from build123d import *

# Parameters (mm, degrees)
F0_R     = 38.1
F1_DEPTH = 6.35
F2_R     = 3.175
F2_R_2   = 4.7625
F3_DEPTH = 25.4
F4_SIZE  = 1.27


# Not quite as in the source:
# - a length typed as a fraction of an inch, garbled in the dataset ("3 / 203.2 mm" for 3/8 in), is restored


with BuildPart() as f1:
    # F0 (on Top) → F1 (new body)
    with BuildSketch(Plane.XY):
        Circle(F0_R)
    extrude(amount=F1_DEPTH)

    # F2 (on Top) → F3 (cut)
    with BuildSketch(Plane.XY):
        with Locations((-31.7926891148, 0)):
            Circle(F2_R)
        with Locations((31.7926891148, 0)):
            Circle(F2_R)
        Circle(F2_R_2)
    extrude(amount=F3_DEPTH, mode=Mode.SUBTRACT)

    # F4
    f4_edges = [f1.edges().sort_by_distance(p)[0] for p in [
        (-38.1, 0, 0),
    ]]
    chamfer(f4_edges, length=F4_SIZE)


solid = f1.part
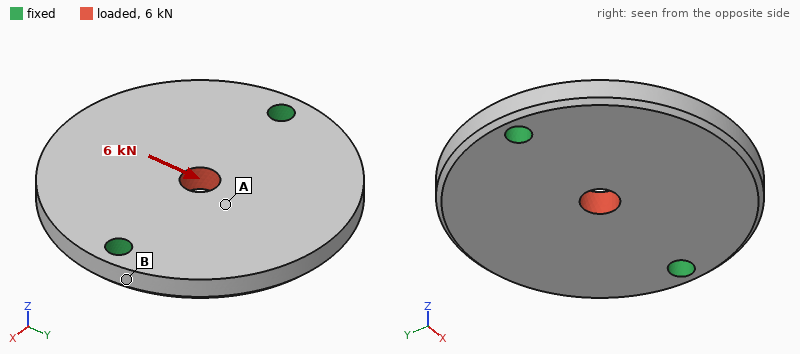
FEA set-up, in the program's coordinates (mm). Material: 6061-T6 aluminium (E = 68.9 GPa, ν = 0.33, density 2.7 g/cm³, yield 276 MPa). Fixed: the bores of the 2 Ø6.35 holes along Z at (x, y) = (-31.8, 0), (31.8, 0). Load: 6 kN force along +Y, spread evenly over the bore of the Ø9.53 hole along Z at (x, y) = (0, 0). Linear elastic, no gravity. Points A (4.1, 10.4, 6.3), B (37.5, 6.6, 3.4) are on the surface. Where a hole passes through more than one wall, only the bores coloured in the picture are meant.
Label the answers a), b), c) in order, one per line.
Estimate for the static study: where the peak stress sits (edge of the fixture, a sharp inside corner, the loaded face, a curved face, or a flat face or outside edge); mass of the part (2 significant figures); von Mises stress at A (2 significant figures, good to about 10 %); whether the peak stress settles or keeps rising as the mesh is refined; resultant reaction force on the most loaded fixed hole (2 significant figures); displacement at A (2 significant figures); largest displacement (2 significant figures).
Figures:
a) edge of the fixture
b) 75 g
c) 23 MPa
d) keeps rising
e) 3.0 kN
f) 13 µm
g) 16 µm
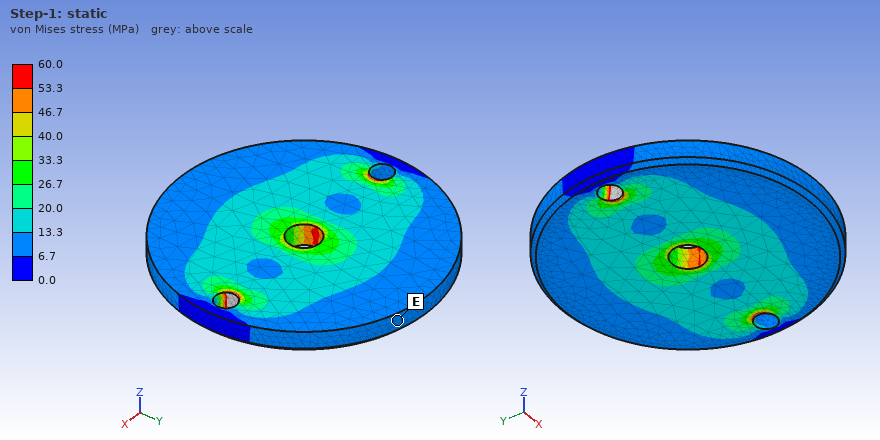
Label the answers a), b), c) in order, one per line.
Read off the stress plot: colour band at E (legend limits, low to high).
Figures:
a) 6.7 to 13.3 MPa
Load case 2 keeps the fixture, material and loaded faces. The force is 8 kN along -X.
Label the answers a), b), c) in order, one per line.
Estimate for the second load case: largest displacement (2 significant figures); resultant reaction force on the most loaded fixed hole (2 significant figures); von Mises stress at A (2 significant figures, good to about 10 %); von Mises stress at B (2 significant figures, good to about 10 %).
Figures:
a) 14 µm
b) 4.0 kN
c) 9.7 MPa
d) 8.9 MPa
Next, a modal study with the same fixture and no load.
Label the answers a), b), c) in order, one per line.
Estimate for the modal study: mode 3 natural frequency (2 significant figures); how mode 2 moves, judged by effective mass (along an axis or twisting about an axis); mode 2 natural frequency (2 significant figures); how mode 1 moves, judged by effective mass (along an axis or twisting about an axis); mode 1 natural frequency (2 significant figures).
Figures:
a) 8800 Hz
b) along Z
c) 4000 Hz
d) twisting about X
e) 3000 Hz
